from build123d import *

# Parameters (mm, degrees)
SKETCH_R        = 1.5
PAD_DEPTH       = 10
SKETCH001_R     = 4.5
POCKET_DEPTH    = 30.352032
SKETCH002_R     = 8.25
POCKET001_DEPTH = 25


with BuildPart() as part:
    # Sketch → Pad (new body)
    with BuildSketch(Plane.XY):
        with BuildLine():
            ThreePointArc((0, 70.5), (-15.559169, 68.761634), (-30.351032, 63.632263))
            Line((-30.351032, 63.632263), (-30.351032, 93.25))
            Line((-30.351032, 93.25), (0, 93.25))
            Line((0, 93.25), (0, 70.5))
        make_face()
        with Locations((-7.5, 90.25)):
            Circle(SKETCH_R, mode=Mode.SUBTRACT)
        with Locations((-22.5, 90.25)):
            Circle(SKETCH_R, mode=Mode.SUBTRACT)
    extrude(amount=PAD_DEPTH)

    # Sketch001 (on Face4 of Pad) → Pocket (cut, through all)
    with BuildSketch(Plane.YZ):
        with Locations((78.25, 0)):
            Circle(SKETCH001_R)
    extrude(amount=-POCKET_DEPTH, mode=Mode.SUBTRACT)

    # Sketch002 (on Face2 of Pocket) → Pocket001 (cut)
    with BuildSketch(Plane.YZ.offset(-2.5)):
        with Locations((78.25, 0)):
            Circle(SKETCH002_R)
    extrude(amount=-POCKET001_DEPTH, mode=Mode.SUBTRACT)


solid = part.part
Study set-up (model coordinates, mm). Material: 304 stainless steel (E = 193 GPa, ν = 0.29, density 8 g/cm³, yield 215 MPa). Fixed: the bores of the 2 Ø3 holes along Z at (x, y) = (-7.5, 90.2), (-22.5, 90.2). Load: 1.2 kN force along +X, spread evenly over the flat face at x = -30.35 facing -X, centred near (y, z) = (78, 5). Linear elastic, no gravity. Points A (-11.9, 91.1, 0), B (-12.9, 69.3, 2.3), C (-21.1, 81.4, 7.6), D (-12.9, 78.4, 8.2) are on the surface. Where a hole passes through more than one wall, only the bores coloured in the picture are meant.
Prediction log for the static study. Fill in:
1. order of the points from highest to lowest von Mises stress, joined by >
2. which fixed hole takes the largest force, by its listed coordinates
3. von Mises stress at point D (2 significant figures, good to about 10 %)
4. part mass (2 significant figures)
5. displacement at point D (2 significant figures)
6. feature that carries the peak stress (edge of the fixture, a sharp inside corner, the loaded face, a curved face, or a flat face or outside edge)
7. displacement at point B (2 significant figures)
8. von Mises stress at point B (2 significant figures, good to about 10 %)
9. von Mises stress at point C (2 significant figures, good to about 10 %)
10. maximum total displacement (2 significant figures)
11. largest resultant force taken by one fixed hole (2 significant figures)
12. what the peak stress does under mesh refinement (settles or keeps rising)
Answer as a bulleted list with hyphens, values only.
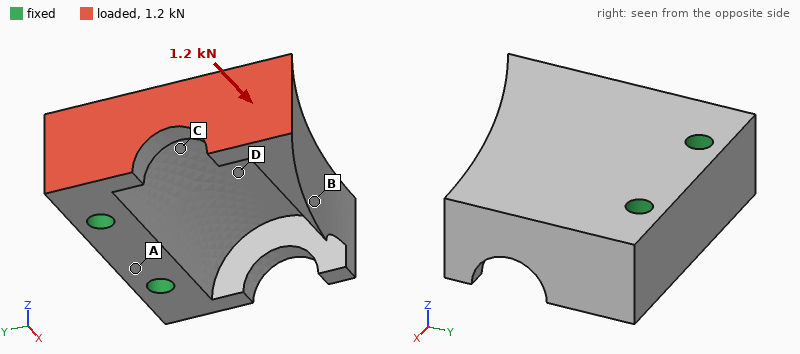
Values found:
- D > C > B > A
- (-22.5, 90.2)
- 42 MPa
- 37 g
- 2.5 µm
- edge of the fixture
- 7.6 µm
- 19 MPa
- 33 MPa
- 14 µm
- 1.1 kN
- keeps rising
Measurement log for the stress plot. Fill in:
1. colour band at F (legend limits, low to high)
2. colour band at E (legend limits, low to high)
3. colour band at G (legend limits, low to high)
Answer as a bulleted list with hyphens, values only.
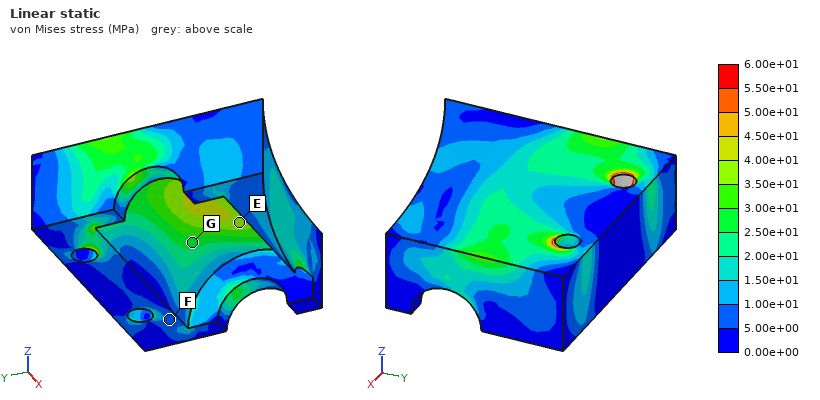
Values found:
- 5.00e+00 to 1.00e+01 MPa
- 3.50e+01 to 4.00e+01 MPa
- 2.50e+01 to 3.00e+01 MPa
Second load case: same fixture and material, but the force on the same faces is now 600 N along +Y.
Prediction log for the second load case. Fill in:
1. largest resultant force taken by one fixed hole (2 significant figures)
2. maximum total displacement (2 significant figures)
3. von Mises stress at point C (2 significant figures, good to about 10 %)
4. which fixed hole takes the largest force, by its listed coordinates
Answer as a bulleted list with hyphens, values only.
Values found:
- 790 N
- 8.9 µm
- 15 MPa
- (-22.5, 90.2)
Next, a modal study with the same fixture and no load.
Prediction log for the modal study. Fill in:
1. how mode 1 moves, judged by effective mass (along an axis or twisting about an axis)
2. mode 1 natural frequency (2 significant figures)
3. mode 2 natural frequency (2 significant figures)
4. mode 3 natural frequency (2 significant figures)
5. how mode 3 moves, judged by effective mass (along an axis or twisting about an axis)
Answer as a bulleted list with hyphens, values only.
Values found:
- along Z
- 6200 Hz
- 12 kHz
- 18 kHz
- along X
